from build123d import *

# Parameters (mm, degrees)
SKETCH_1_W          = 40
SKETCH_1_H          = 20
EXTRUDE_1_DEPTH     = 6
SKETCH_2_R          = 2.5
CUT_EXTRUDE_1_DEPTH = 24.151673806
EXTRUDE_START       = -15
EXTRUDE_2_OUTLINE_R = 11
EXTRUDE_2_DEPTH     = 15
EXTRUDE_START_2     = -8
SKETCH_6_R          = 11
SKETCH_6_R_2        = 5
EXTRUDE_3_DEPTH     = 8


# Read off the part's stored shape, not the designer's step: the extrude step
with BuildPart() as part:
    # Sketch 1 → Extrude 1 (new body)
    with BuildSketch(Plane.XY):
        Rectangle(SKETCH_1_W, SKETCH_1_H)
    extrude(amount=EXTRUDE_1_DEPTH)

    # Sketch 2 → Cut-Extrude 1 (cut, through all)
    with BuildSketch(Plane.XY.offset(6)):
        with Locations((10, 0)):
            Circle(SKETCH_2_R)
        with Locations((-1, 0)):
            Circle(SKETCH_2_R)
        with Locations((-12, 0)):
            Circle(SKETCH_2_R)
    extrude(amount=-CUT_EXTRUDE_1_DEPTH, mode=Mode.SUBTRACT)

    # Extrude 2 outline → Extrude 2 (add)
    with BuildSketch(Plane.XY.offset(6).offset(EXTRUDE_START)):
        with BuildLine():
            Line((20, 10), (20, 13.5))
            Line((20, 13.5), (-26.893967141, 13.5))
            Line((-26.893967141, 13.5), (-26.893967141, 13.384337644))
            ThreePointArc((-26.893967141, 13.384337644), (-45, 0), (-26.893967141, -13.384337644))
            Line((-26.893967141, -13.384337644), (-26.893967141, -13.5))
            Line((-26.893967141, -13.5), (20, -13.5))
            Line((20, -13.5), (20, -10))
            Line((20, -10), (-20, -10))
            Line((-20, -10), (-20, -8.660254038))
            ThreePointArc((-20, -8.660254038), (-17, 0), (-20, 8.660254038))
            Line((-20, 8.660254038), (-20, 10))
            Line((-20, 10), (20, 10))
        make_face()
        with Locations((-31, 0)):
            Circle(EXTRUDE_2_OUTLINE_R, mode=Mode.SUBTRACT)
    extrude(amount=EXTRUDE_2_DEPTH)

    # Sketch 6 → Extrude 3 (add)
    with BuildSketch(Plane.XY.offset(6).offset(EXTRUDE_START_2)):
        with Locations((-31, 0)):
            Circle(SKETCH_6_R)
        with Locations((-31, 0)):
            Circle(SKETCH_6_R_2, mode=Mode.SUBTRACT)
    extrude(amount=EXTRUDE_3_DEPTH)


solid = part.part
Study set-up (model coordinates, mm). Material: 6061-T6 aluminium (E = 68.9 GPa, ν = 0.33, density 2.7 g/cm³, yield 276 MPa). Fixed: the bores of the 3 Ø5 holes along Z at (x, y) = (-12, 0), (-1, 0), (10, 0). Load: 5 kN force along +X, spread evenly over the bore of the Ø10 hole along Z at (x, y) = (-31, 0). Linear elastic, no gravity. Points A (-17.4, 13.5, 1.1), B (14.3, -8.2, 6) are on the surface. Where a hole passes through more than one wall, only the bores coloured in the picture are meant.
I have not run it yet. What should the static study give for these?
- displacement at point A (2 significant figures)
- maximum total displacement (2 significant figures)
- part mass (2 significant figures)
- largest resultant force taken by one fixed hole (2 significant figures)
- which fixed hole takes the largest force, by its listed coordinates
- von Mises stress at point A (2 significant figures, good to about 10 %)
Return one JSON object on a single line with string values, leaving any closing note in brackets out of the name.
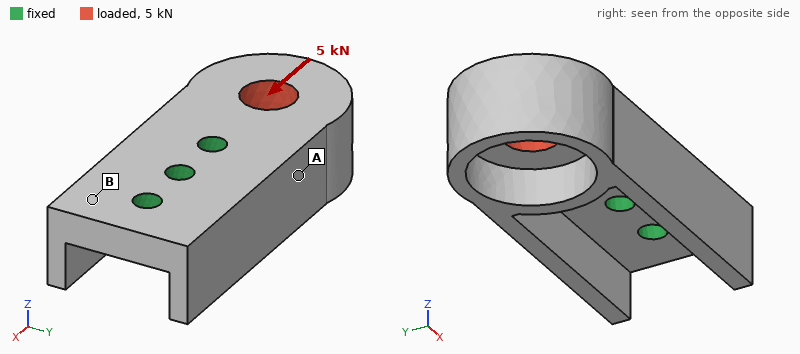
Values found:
{"displacement at point A": "6.3 µm", "maximum total displacement": "16 µm", "part mass": "40 g", "largest resultant force taken by one fixed hole": "3.4 kN", "which fixed hole takes the largest force, by its listed coordinates": "(-12, 0)", "von Mises stress at point A": "15 MPa"}
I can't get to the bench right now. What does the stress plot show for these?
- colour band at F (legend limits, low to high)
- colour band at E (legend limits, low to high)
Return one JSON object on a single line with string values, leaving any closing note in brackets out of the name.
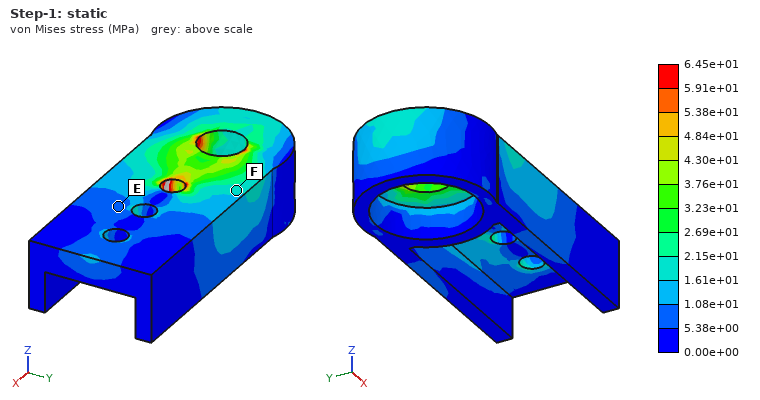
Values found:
{"colour band at F": "1.61e+01 to 2.15e+01 MPa", "colour band at E": "5.38e+00 to 1.08e+01 MPa"}
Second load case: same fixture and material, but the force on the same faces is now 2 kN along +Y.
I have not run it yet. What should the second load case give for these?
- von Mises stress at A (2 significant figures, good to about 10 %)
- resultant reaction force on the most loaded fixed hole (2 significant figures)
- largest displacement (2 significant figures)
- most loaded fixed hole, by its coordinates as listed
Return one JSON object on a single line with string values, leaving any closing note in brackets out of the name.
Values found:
{"von Mises stress at A": "28 MPa", "resultant reaction force on the most loaded fixed hole": "3.4 kN", "largest displacement": "43 µm", "most loaded fixed hole, by its coordinates as listed": "(-12, 0)"}
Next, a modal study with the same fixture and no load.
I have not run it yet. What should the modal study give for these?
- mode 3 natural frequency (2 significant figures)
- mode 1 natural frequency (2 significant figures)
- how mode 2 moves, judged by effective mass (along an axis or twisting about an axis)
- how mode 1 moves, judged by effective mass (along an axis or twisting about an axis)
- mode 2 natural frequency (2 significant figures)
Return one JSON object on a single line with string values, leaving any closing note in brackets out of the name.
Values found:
{"mode 3 natural frequency": "10 kHz", "mode 1 natural frequency": "6300 Hz", "how mode 2 moves, judged by effective mass": "along Y", "how mode 1 moves, judged by effective mass": "along Z", "mode 2 natural frequency": "8300 Hz"}
